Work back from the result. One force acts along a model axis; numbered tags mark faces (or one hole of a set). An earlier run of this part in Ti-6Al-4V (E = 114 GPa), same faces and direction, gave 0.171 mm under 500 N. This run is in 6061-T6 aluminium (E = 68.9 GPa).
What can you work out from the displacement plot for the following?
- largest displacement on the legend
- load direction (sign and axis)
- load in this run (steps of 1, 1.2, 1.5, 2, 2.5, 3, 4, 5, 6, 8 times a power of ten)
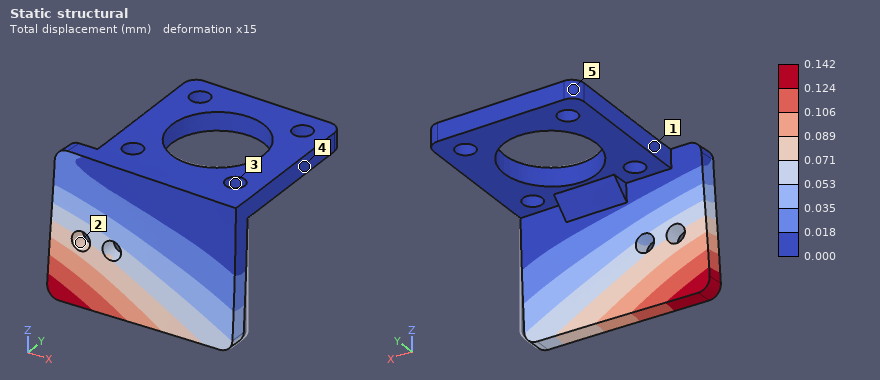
0.142 mm
-Y
250 N
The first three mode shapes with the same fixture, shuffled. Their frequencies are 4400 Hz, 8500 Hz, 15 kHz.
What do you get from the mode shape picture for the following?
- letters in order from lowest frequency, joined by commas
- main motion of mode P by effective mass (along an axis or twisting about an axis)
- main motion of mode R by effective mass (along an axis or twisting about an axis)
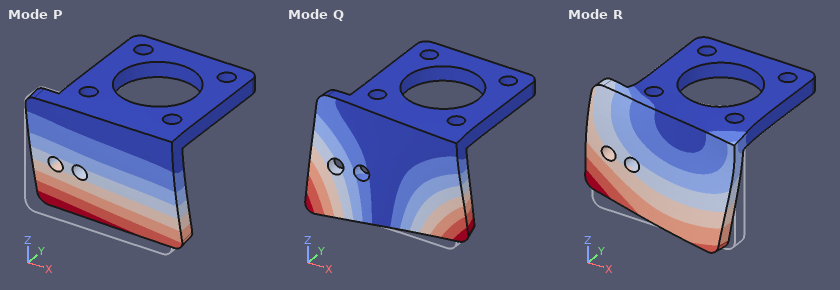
P, Q, R
along Y
along X
